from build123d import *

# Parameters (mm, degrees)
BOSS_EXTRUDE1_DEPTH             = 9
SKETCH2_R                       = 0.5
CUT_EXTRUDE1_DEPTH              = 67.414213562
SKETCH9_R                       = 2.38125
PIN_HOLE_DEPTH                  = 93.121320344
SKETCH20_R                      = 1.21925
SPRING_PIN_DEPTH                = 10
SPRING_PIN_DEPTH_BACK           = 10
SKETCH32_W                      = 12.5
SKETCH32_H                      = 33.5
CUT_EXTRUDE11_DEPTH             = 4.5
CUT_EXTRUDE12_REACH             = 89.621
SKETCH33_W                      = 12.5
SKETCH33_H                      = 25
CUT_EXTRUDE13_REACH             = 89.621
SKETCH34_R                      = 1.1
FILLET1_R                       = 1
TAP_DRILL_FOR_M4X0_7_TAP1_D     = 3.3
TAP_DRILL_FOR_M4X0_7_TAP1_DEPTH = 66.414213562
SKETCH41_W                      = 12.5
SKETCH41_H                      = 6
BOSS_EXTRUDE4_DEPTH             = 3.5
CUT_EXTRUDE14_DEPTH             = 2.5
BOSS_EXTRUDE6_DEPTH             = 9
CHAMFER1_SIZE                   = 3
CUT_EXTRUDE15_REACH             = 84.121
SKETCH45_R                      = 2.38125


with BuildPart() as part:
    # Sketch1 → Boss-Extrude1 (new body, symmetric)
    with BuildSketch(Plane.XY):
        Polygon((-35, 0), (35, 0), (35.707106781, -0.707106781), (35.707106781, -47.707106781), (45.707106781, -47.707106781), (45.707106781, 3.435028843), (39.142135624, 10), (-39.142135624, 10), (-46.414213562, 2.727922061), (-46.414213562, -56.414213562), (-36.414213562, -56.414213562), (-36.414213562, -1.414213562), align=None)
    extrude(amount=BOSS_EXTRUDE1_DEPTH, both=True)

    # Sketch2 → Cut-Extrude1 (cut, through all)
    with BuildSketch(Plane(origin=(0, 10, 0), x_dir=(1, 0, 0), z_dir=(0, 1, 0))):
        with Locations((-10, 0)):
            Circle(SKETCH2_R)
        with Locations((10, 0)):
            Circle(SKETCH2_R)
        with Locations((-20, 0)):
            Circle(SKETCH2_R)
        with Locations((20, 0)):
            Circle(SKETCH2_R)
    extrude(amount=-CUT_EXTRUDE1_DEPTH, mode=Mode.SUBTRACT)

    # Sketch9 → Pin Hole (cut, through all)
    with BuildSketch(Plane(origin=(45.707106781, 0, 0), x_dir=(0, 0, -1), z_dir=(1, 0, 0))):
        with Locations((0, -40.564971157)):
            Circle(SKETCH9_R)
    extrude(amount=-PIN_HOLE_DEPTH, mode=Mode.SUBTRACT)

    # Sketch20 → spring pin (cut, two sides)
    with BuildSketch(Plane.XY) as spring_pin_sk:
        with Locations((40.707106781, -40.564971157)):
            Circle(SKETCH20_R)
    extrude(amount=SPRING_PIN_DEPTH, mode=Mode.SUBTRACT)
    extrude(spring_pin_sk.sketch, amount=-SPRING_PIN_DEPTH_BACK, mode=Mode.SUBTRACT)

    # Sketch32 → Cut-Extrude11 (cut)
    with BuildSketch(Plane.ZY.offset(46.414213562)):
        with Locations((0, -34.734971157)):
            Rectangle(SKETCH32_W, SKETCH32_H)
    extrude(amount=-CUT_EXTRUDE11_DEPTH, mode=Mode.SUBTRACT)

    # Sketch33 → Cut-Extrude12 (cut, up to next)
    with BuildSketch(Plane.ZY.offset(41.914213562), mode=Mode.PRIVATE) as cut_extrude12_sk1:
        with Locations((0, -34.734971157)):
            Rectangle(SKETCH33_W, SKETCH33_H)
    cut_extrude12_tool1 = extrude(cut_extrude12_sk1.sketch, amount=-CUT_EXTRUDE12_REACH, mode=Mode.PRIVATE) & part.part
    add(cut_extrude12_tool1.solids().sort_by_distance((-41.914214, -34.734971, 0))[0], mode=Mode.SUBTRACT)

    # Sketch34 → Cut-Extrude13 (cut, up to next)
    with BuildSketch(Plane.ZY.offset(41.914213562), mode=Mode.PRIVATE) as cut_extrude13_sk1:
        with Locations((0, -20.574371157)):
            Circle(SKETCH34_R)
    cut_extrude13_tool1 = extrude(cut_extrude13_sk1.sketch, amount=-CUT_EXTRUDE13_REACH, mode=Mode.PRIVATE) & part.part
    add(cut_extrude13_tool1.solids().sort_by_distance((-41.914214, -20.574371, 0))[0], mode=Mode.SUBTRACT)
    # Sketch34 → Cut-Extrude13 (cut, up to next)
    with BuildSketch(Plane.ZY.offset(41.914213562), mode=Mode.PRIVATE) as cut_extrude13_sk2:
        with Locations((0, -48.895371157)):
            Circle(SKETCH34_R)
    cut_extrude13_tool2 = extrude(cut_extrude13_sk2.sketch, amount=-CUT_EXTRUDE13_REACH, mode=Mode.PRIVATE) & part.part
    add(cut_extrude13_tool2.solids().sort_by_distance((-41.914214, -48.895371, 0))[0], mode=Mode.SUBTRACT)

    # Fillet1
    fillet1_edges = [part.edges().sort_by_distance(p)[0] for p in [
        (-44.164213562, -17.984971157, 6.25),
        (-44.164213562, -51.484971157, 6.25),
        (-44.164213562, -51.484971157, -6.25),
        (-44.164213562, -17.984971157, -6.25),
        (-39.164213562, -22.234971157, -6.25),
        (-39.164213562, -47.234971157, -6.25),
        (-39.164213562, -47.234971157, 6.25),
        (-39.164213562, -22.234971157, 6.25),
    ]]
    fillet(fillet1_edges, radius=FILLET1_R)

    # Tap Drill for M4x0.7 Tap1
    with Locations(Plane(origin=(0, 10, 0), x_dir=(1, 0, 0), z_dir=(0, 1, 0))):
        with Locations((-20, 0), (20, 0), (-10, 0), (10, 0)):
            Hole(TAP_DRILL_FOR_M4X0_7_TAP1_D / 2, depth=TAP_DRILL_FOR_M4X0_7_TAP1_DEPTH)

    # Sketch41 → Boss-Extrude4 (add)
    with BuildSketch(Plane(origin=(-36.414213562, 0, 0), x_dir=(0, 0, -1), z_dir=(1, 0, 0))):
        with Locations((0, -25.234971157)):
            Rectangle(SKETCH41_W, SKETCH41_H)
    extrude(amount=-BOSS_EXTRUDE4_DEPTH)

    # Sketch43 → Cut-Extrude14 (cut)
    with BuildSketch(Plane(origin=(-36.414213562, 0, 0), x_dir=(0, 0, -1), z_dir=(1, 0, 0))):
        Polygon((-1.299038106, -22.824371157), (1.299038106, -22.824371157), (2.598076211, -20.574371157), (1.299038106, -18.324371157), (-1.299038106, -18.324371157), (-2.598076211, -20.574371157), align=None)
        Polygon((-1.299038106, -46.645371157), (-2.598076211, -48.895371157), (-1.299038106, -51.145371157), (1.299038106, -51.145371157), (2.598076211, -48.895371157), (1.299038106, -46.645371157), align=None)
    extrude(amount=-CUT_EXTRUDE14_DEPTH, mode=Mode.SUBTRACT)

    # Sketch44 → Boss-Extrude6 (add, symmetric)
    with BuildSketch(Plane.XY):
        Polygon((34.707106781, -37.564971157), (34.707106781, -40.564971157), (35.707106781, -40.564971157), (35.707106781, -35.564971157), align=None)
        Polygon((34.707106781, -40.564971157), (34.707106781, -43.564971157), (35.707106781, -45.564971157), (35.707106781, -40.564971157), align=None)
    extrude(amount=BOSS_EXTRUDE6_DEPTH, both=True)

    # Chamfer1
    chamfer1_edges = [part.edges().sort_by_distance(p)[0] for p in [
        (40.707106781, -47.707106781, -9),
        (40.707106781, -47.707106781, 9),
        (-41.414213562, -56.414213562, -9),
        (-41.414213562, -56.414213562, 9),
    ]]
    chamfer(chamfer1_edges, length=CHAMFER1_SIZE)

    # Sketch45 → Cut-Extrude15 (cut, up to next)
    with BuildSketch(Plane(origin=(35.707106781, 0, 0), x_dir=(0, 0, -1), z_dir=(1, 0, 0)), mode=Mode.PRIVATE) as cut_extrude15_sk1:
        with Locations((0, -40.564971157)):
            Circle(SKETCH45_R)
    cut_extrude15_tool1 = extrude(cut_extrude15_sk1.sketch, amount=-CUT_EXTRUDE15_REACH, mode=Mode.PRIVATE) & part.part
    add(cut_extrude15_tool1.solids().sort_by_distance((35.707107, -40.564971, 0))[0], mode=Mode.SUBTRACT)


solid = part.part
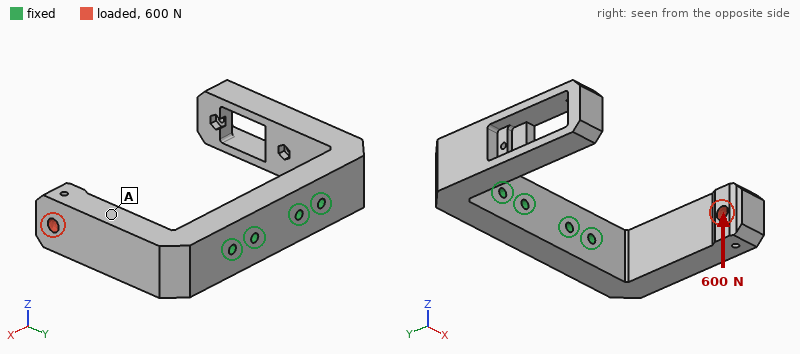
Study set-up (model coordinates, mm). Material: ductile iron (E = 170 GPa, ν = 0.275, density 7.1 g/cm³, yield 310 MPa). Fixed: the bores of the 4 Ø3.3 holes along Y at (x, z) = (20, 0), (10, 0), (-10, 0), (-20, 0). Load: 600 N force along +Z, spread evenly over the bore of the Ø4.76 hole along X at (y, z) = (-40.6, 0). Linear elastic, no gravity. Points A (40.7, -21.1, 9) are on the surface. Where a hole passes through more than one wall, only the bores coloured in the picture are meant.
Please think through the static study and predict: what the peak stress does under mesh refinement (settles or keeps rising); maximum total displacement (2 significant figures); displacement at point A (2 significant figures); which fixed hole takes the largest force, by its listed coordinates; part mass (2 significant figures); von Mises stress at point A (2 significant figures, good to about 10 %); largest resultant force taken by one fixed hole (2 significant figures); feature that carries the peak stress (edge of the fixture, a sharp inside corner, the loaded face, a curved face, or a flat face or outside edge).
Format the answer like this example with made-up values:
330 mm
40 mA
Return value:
keeps rising
0.14 mm
0.068 mm
(20, 0)
220 g
22 MPa
1.2 kN
edge of the fixture
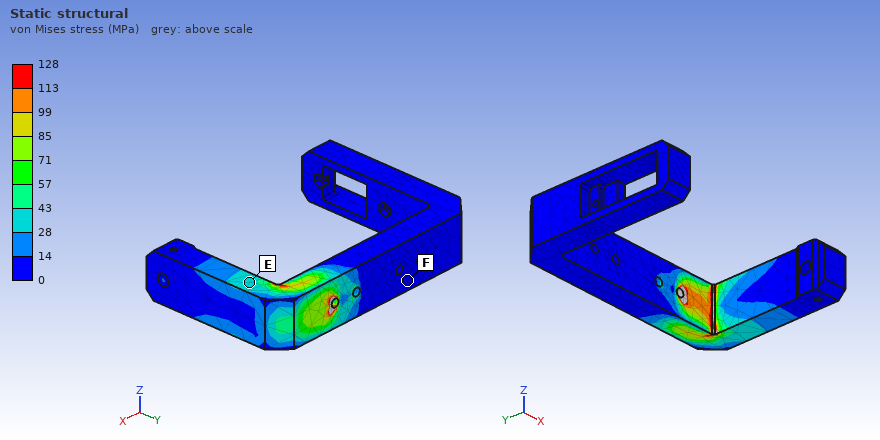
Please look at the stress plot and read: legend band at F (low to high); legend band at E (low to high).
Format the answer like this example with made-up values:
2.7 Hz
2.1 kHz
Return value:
0 to 14 MPa
28 to 43 MPa
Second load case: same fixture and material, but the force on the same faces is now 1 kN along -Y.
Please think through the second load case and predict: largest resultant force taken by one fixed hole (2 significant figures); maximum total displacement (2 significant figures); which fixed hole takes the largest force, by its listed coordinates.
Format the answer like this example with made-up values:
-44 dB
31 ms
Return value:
1.4 kN
51 µm
(20, 0)
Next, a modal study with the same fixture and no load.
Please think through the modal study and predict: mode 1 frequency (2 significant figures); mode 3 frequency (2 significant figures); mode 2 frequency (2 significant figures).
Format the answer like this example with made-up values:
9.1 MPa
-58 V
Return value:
1700 Hz
1800 Hz
1800 Hz
